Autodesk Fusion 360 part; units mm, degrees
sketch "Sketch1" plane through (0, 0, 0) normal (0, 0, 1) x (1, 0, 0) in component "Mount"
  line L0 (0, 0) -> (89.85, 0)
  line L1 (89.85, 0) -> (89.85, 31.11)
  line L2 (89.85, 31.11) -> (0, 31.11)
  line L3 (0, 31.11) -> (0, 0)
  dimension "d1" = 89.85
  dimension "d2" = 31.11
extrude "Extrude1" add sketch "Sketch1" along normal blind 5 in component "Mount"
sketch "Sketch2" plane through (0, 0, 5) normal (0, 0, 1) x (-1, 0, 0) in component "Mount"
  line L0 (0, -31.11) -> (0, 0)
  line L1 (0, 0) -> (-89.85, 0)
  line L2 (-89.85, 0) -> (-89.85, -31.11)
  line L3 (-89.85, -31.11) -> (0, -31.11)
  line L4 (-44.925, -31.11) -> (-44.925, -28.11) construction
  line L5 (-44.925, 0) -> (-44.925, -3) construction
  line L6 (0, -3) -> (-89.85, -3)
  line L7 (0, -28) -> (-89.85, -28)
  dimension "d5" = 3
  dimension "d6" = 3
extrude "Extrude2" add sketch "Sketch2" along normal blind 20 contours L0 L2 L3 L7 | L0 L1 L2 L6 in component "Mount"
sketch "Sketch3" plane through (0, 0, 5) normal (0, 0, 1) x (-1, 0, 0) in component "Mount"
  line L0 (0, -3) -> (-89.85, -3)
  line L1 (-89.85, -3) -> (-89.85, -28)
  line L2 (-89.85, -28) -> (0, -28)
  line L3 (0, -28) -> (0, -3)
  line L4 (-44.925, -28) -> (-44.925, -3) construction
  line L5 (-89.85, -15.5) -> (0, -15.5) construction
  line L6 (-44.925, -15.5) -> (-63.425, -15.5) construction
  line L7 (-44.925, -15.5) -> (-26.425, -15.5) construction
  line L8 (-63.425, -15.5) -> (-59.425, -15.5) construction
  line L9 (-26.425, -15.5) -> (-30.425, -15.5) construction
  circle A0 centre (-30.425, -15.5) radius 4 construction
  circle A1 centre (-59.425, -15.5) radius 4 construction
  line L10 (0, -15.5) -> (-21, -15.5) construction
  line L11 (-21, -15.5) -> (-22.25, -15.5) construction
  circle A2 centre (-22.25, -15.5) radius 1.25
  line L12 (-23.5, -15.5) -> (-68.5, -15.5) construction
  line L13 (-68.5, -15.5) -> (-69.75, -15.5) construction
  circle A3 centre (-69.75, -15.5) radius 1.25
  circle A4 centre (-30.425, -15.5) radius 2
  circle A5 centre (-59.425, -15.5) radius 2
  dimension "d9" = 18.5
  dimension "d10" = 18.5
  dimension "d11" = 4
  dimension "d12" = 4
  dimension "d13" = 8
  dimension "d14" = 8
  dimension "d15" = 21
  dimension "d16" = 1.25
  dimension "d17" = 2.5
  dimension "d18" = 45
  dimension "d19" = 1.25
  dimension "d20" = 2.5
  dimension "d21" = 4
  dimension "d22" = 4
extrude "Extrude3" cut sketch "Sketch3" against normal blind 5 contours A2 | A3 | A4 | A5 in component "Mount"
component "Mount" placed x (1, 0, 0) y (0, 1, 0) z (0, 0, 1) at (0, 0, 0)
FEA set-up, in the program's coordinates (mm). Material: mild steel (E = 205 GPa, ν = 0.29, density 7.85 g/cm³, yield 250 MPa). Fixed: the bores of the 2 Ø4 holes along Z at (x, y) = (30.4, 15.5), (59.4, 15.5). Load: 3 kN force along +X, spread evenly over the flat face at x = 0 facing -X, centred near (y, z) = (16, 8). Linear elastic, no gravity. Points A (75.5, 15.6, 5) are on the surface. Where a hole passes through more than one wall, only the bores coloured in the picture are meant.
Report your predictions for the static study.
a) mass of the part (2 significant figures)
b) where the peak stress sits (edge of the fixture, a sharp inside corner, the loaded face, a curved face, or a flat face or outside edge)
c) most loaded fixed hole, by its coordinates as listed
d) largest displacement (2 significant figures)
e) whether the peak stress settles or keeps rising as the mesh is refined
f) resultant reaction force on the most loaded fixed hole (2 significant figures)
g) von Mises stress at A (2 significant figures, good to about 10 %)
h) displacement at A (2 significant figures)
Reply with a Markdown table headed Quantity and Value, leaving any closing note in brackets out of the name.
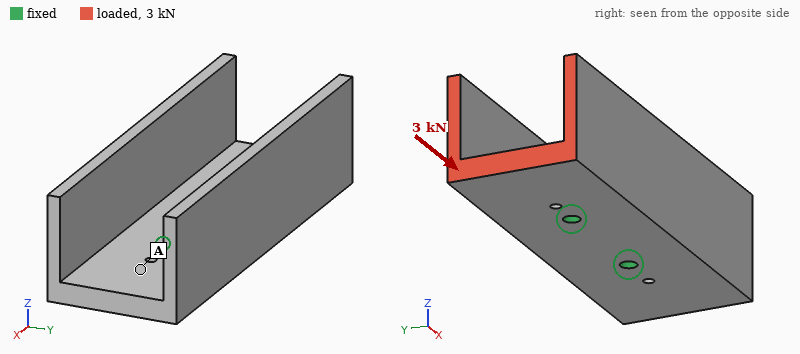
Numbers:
| Quantity | Value |
|---|---|
| mass of the part | 190 g |
| where the peak stress sits | edge of the fixture |
| most loaded fixed hole, by its coordinates as listed | (30.4, 15.5) |
| largest displacement | 12 µm |
| whether the peak stress settles or keeps rising as the mesh is refined | keeps rising |
| resultant reaction force on the most loaded fixed hole | 2.0 kN |
| von Mises stress at A | 7.2 MPa |
| displacement at A | 3.7 µm |
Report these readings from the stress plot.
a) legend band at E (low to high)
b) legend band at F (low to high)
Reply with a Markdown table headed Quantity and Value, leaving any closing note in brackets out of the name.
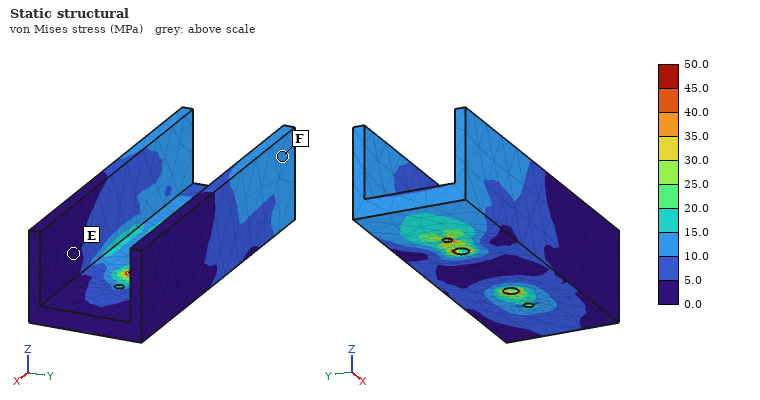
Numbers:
| Quantity | Value |
|---|---|
| legend band at E | 0.0 to 5.0 MPa |
| legend band at F | 10.0 to 15.0 MPa |
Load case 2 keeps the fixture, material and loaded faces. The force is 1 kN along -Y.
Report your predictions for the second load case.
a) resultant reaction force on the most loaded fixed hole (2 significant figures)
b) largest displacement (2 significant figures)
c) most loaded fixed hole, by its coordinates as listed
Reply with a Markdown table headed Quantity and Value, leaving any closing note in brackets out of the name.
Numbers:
| Quantity | Value |
|---|---|
| resultant reaction force on the most loaded fixed hole | 1.9 kN |
| largest displacement | 69 µm |
| most loaded fixed hole, by its coordinates as listed | (30.4, 15.5) |
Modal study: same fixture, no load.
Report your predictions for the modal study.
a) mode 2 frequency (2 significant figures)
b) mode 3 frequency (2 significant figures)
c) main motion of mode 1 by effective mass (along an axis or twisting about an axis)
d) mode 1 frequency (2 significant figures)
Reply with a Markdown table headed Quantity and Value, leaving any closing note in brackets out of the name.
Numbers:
| Quantity | Value |
|---|---|
| mode 2 frequency | 3500 Hz |
| mode 3 frequency | 4200 Hz |
| main motion of mode 1 by effective mass | along Y |
| mode 1 frequency | 3300 Hz |
